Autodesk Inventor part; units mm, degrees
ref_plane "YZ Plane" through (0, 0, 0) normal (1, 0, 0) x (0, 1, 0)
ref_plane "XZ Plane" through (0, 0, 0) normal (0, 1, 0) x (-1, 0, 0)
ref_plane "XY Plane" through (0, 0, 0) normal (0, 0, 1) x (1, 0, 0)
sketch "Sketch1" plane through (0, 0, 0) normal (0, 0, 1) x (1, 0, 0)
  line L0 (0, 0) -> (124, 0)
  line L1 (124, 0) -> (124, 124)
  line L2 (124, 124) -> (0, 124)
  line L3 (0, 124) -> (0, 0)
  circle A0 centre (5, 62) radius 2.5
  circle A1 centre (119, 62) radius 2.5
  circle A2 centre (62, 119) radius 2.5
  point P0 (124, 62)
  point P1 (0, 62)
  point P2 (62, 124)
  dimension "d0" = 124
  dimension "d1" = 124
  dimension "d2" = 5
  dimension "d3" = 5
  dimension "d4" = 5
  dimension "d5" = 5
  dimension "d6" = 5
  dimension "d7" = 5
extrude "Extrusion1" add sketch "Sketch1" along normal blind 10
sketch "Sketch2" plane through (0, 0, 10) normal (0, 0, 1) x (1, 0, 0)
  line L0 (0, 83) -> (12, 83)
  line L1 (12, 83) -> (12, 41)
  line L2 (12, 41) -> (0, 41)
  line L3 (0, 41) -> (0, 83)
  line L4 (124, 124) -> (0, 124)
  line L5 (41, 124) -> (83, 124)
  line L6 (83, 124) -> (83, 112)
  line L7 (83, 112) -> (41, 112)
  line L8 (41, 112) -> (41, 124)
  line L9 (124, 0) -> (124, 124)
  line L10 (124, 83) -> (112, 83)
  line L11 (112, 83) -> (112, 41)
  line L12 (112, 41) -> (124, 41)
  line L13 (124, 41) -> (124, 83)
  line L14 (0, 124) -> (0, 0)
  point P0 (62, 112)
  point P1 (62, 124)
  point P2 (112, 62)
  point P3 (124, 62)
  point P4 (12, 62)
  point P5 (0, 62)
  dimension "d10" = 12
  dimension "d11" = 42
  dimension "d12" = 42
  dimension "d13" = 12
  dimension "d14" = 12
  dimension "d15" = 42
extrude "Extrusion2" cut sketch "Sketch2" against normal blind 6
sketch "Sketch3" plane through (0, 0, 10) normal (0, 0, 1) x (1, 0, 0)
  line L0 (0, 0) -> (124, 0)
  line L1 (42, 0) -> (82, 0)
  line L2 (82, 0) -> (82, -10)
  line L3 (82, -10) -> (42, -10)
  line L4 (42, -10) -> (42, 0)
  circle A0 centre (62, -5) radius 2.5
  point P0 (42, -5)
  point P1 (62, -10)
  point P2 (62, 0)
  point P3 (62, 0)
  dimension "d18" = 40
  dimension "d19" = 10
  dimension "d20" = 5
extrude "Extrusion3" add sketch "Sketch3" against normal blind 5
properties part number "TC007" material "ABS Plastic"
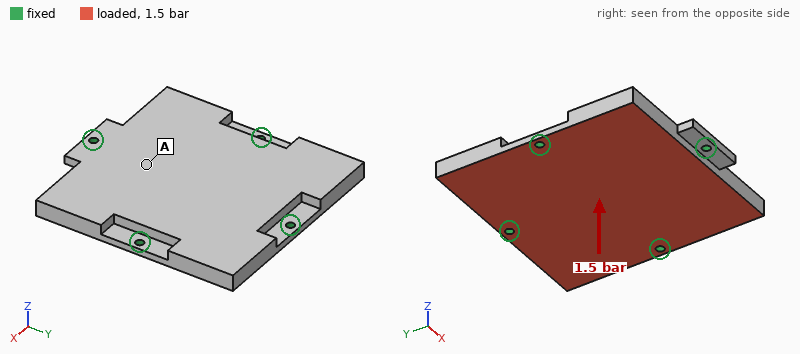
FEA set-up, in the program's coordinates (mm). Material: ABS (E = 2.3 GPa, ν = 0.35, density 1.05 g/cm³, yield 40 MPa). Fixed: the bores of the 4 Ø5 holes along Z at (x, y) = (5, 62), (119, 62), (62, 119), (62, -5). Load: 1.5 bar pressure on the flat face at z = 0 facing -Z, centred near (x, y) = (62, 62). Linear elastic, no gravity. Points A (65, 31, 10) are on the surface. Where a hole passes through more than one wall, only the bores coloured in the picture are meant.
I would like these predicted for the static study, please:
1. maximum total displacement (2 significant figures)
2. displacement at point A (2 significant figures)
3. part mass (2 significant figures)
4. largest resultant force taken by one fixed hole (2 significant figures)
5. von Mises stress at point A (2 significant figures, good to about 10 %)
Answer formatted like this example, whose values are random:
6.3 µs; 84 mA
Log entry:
0.70 mm; 0.45 mm; 150 g; 760 N; 3.4 MPa
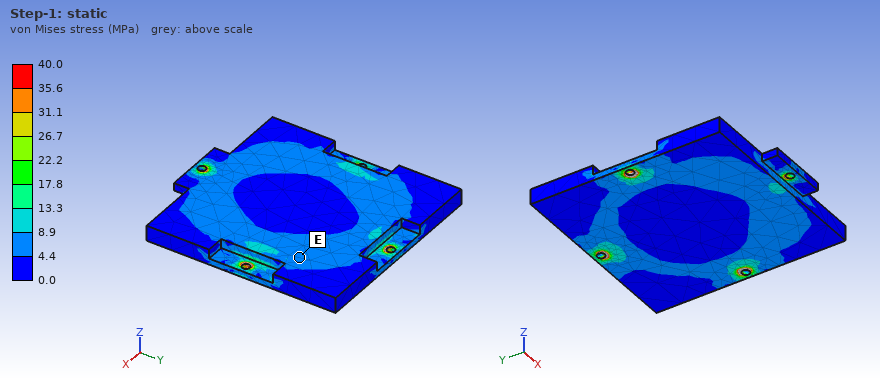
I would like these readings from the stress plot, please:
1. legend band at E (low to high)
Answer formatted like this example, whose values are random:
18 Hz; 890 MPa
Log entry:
4.4 to 8.9 MPa
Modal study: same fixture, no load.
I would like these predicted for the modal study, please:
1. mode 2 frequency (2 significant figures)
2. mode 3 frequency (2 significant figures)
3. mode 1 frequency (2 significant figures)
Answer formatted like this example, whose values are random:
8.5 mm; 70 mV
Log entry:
800 Hz; 800 Hz; 700 Hz
